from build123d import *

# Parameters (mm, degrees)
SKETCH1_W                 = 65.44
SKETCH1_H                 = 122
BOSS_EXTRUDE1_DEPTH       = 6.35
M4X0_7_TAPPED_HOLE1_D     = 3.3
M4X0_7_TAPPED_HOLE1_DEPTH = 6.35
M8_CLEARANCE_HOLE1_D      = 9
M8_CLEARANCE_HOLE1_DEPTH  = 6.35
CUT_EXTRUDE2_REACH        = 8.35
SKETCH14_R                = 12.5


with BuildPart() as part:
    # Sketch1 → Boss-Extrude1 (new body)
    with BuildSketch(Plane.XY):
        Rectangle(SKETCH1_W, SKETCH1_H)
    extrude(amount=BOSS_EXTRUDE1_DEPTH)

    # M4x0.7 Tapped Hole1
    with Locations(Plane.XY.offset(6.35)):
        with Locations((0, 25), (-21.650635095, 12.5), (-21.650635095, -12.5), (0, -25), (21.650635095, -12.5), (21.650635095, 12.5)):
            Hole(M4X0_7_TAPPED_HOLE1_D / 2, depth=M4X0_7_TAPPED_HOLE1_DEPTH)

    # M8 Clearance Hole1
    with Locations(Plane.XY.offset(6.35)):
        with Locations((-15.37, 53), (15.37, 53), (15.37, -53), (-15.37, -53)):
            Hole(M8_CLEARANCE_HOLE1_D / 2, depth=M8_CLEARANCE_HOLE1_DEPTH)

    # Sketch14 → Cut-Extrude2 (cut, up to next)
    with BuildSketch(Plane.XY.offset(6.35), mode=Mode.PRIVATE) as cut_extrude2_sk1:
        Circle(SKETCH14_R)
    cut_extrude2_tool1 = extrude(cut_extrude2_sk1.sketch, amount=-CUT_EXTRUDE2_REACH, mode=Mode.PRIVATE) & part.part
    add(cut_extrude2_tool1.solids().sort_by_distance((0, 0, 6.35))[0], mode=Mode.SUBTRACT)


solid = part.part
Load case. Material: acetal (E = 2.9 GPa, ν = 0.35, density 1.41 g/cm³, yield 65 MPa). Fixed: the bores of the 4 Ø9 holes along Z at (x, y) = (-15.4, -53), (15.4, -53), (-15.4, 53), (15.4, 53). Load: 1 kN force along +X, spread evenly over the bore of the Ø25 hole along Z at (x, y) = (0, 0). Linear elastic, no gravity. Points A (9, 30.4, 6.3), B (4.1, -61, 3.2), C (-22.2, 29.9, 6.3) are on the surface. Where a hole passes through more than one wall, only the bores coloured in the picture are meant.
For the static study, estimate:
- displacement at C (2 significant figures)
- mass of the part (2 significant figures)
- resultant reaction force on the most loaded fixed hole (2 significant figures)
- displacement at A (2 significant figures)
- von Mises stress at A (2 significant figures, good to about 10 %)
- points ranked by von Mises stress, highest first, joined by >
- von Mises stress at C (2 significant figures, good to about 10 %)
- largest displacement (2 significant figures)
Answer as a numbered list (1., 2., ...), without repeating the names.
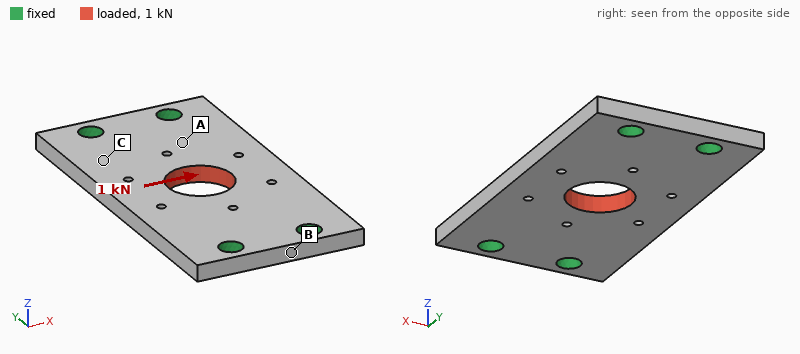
1. 43 µm
2. 64 g
3. 340 N
4. 39 µm
5. 2.9 MPa
6. A > C > B
7. 1.6 MPa
8. 90 µm
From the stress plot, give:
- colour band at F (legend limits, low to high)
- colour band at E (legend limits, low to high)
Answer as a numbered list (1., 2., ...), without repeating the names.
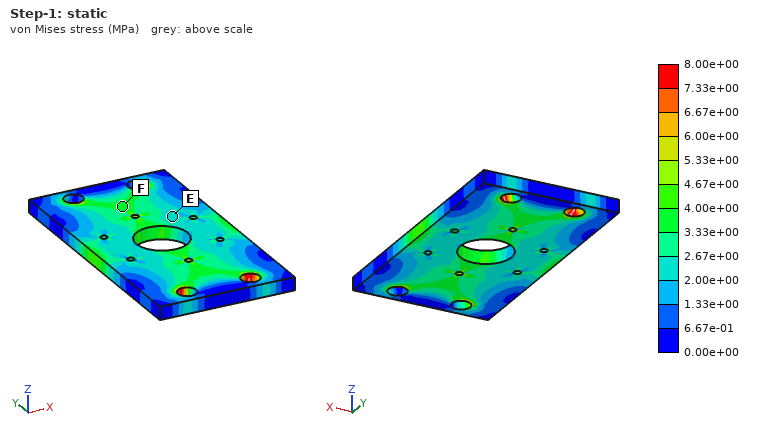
1. 3.33e+00 to 4.00e+00 MPa
2. 2.00e+00 to 2.67e+00 MPa
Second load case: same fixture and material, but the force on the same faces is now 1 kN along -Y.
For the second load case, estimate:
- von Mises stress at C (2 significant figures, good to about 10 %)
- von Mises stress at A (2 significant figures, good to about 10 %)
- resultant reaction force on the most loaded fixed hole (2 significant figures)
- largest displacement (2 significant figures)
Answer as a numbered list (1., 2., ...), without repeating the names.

1. 1.1 MPa
2. 1.9 MPa
3. 250 N
4. 29 µm
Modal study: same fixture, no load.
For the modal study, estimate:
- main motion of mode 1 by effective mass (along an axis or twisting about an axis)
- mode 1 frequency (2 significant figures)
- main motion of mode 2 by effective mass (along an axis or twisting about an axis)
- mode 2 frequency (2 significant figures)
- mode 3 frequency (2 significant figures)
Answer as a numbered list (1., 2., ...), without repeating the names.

1. along Z
2. 900 Hz
3. twisting about Y
4. 1100 Hz
5. 2200 Hz
